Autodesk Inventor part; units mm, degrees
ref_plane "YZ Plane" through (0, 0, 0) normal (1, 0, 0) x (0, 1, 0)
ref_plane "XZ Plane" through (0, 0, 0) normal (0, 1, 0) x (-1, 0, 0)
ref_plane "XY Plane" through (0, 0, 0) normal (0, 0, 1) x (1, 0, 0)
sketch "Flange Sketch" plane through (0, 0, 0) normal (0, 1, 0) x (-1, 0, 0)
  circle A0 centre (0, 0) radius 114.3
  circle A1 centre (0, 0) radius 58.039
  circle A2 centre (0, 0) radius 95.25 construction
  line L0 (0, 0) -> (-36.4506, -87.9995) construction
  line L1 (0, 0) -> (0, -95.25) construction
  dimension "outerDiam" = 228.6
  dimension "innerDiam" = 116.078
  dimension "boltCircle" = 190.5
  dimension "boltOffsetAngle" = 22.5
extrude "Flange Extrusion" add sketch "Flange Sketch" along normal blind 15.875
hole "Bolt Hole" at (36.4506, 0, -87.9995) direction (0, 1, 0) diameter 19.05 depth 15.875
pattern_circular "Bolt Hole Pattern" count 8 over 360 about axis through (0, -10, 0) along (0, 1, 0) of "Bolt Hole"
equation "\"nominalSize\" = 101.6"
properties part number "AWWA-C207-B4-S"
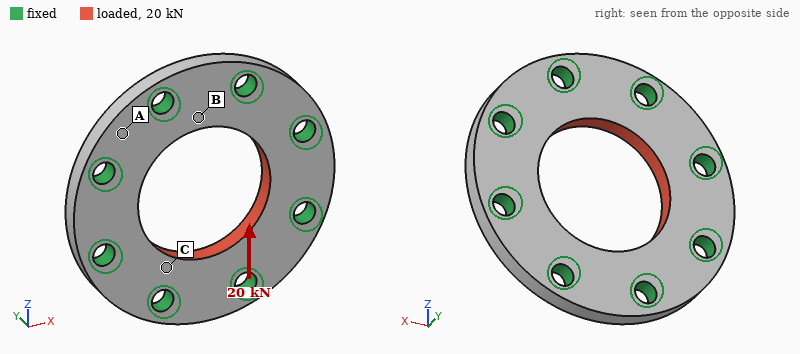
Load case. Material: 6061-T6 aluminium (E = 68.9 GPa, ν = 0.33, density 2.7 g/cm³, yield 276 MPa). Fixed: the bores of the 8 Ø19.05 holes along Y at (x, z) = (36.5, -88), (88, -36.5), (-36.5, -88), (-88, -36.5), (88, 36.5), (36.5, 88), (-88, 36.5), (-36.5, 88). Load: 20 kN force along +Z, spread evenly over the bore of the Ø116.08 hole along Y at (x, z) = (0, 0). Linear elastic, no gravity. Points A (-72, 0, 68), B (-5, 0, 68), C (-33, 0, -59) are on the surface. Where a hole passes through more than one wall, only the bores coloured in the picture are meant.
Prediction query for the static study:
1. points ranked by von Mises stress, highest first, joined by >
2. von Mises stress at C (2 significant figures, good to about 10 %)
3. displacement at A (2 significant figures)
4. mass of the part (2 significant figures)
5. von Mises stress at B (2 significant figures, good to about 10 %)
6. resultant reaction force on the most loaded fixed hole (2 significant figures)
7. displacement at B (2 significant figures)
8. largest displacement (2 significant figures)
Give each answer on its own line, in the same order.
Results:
C > B > A
4.6 MPa
0.99 µm
1.2 kg
2.8 MPa
3.3 kN
2.1 µm
2.8 µm
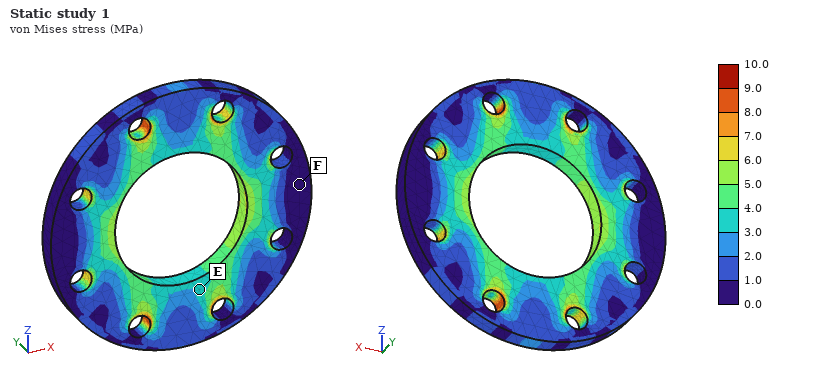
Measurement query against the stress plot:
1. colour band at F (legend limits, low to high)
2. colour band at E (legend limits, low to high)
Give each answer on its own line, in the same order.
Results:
0.0 to 1.0 MPa
3.0 to 4.0 MPa
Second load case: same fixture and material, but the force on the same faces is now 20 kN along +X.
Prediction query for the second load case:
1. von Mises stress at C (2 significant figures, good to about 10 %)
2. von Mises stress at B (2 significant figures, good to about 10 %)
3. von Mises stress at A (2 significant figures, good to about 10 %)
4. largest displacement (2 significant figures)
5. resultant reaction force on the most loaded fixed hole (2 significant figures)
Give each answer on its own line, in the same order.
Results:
3.0 MPa
4.4 MPa
0.76 MPa
2.8 µm
3.3 kN
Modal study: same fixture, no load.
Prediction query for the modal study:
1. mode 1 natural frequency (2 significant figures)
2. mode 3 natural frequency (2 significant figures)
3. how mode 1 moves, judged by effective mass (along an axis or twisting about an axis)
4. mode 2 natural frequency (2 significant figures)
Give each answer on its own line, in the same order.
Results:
10 kHz
11 kHz
along Y
11 kHz
